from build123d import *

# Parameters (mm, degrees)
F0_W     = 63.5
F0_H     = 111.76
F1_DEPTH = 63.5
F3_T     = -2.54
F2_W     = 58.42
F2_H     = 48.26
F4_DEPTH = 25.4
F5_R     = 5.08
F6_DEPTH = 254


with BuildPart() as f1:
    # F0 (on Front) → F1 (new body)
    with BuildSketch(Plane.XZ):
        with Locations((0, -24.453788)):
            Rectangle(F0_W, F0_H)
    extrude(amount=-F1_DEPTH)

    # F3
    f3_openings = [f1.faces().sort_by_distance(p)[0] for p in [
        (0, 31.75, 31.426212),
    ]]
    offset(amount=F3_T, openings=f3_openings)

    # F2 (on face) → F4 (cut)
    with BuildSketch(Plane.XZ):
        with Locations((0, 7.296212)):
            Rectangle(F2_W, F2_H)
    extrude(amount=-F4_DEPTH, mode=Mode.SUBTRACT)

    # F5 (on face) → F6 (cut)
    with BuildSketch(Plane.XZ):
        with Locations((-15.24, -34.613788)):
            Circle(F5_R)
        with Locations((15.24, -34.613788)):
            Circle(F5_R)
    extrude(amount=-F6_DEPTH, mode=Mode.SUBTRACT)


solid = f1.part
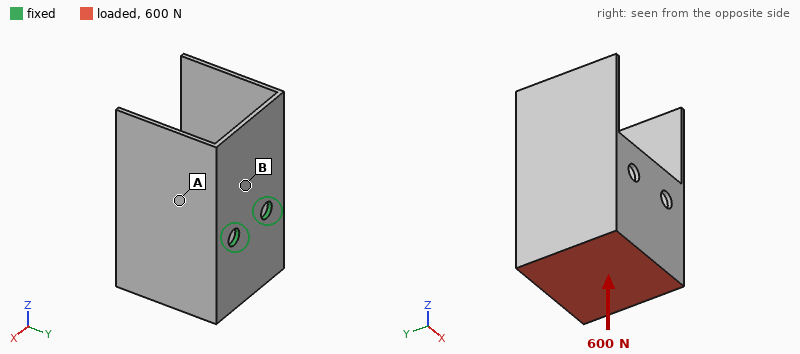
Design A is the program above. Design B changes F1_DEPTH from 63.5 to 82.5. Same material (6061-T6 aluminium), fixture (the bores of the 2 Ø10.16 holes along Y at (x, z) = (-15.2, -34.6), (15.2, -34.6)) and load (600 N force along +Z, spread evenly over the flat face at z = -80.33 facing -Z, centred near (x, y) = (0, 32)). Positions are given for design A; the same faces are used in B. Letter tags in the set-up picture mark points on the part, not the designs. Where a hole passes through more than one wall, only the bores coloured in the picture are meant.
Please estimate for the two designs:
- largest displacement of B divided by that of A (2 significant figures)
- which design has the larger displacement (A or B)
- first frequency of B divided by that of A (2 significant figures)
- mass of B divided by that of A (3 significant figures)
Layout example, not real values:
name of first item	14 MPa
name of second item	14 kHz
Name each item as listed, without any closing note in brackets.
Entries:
largest displacement of B divided by that of A	1.5
which design has the larger displacement	B
first frequency of B divided by that of A	0.77
mass of B divided by that of A	1.19
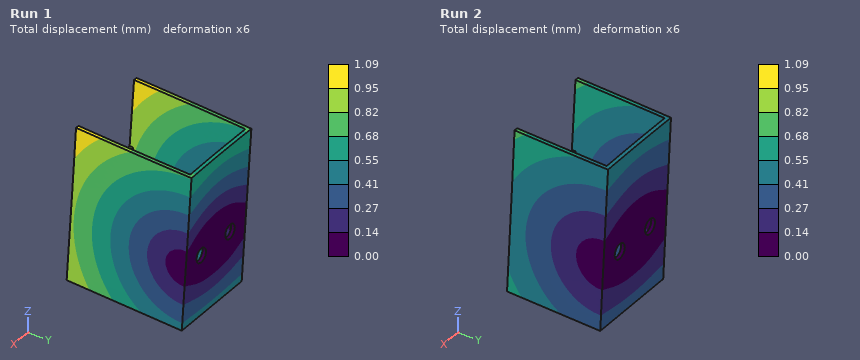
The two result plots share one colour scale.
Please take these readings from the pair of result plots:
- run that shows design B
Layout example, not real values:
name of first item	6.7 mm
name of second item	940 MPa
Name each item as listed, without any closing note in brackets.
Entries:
run that shows design B	Run 1
